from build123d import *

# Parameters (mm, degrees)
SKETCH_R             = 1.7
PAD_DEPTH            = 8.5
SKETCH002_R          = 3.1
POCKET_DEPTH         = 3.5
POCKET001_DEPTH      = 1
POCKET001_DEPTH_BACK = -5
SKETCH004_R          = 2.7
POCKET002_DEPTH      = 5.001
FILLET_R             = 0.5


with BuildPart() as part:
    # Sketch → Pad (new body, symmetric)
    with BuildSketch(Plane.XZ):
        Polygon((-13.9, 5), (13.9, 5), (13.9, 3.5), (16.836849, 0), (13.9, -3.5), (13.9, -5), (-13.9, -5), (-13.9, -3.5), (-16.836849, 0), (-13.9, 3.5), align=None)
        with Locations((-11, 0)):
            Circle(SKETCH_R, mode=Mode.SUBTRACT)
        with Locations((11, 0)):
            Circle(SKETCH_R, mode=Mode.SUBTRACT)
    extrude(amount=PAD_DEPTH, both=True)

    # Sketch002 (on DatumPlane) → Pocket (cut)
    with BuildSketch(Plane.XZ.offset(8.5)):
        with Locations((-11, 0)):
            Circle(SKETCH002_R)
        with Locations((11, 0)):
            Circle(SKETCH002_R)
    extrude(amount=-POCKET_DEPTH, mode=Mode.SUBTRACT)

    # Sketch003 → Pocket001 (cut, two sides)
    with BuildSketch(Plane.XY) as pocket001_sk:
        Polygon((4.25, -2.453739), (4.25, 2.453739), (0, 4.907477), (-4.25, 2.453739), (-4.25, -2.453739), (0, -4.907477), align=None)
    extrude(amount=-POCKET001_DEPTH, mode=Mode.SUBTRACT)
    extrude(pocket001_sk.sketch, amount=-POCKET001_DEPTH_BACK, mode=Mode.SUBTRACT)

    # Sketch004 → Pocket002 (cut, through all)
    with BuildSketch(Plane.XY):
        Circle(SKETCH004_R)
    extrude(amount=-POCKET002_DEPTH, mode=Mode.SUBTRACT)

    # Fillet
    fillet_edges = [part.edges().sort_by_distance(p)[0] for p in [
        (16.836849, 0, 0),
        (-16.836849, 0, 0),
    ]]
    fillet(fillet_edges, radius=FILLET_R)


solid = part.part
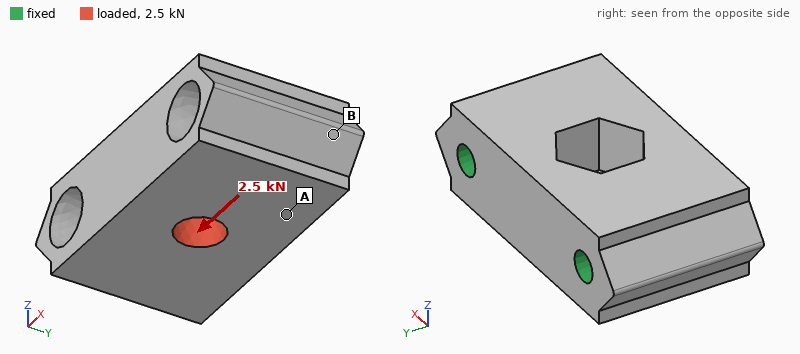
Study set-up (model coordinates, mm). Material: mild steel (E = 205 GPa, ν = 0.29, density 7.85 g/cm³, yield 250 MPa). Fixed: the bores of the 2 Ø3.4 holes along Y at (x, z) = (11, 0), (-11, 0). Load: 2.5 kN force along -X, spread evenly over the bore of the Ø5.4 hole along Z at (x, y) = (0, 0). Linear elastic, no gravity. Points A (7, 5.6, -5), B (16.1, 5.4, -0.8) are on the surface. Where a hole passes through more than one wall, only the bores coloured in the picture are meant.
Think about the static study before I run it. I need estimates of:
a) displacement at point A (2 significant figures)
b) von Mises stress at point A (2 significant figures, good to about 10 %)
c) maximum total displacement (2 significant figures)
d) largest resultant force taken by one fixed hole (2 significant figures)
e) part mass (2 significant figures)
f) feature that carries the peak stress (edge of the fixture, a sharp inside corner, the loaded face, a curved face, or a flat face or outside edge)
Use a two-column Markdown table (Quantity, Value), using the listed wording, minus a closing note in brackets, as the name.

| Quantity | Value |
|---|---|
| displacement at point A | 0.33 µm |
| von Mises stress at point A | 12 MPa |
| maximum total displacement | 1.3 µm |
| largest resultant force taken by one fixed hole | 1.3 kN |
| part mass | 33 g |
| feature that carries the peak stress | a sharp inside corner |
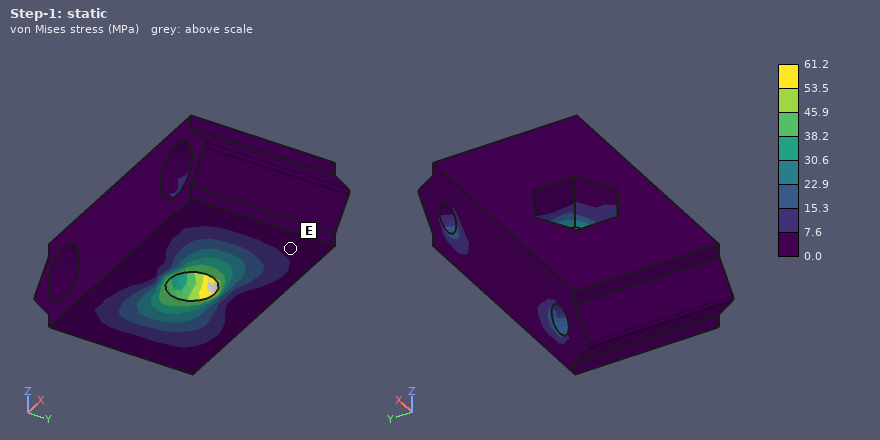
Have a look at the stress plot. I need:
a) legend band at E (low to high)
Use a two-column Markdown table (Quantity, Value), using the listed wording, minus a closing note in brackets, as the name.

| Quantity | Value |
|---|---|
| legend band at E | 0.0 to 7.6 MPa |
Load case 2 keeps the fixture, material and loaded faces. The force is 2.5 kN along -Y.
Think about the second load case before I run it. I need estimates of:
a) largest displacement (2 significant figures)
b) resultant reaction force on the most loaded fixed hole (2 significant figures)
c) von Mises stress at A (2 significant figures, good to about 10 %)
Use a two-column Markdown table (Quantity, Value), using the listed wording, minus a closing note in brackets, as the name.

| Quantity | Value |
|---|---|
| largest displacement | 2.7 µm |
| resultant reaction force on the most loaded fixed hole | 1.3 kN |
| von Mises stress at A | 26 MPa |
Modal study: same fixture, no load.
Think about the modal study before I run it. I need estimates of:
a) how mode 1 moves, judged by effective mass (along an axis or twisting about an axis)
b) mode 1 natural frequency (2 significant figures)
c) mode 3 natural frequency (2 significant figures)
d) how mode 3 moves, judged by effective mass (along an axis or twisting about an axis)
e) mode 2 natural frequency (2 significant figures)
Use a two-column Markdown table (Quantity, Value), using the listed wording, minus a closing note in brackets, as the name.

| Quantity | Value |
|---|---|
| how mode 1 moves, judged by effective mass | along Z |
| mode 1 natural frequency | 46 kHz |
| mode 3 natural frequency | 67 kHz |
| how mode 3 moves, judged by effective mass | along Y |
| mode 2 natural frequency | 59 kHz |
